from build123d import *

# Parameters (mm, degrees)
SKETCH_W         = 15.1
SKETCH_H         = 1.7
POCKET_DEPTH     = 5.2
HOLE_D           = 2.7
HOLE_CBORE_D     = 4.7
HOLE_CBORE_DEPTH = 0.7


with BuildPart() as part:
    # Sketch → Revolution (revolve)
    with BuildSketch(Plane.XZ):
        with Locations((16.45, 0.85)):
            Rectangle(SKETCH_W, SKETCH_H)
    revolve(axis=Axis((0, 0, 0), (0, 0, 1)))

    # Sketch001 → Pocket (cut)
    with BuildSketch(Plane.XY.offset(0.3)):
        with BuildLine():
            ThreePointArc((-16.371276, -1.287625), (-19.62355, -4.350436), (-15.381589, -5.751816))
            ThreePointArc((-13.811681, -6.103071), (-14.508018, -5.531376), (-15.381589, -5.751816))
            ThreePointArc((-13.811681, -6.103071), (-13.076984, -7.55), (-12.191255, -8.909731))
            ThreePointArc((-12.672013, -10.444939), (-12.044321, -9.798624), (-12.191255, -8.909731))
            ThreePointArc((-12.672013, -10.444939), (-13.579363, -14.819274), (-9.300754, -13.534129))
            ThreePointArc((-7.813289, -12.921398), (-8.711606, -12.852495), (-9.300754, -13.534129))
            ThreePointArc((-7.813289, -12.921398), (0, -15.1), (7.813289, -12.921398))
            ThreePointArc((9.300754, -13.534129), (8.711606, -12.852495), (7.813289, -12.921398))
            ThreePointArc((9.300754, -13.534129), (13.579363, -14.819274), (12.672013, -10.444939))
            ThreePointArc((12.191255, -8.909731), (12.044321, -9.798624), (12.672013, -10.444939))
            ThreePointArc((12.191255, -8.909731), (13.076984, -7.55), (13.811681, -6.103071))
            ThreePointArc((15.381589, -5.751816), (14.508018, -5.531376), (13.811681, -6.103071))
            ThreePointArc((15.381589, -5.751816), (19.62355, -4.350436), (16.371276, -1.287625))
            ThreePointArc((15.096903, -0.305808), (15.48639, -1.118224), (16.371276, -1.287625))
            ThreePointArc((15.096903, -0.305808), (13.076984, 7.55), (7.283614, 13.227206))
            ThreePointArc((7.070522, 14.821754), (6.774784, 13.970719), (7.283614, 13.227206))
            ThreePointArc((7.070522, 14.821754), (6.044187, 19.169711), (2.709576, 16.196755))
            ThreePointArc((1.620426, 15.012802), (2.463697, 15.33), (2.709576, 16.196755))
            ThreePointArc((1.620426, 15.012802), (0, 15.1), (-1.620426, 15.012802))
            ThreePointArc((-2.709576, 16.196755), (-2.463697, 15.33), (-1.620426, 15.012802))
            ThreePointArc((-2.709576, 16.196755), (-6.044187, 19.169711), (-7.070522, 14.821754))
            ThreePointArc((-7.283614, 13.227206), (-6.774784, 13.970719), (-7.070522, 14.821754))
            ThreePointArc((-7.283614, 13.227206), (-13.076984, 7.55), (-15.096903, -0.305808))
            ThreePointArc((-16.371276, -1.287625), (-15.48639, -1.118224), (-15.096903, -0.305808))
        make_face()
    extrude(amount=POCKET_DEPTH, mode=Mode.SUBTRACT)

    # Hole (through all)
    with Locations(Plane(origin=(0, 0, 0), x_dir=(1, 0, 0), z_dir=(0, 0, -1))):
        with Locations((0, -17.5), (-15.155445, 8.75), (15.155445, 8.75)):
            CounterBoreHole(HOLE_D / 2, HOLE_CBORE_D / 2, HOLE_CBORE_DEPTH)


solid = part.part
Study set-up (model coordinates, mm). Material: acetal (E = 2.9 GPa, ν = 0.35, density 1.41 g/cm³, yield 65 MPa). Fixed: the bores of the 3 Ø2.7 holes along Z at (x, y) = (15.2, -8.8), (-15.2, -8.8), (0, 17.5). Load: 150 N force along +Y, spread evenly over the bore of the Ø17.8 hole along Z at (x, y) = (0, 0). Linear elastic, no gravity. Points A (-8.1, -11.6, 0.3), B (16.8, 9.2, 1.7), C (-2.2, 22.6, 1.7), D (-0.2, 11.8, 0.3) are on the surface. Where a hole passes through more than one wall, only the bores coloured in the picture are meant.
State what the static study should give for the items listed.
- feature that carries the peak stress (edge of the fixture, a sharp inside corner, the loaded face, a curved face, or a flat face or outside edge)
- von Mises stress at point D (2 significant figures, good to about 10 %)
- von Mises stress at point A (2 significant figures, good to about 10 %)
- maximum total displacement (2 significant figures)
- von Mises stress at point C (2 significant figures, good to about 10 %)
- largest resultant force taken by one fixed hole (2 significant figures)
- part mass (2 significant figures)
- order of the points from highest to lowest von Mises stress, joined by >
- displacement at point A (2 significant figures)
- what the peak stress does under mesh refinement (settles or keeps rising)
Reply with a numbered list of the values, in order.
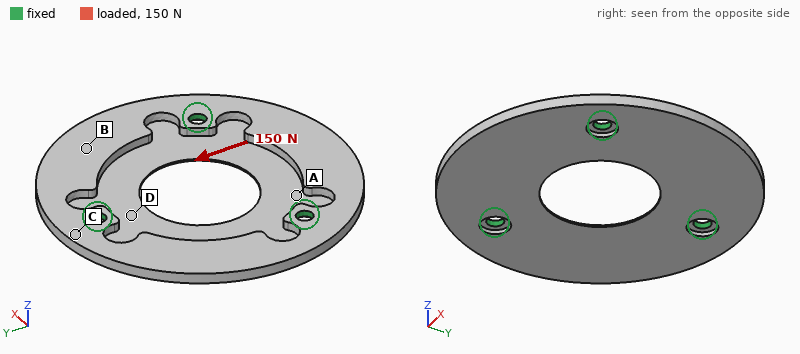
1. a sharp inside corner
2. 10 MPa
3. 7.3 MPa
4. 0.25 mm
5. 4.6 MPa
6. 52 N
7. 2.5 g
8. D > A > C > B
9. 0.067 mm
10. keeps rising
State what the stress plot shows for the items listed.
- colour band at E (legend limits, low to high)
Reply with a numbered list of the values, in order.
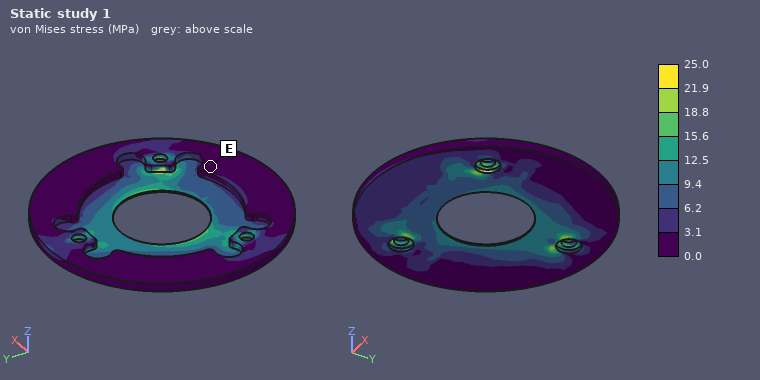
1. 0.0 to 3.1 MPa
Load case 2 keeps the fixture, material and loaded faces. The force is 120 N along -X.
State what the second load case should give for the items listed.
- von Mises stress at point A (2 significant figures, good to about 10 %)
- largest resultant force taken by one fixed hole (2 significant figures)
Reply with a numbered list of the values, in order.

1. 6.2 MPa
2. 42 N
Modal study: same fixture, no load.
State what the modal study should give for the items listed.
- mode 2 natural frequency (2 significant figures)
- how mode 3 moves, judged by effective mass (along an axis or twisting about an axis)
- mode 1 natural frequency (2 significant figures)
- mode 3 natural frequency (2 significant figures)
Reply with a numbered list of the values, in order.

1. 940 Hz
2. along Z
3. 940 Hz
4. 1100 Hz
